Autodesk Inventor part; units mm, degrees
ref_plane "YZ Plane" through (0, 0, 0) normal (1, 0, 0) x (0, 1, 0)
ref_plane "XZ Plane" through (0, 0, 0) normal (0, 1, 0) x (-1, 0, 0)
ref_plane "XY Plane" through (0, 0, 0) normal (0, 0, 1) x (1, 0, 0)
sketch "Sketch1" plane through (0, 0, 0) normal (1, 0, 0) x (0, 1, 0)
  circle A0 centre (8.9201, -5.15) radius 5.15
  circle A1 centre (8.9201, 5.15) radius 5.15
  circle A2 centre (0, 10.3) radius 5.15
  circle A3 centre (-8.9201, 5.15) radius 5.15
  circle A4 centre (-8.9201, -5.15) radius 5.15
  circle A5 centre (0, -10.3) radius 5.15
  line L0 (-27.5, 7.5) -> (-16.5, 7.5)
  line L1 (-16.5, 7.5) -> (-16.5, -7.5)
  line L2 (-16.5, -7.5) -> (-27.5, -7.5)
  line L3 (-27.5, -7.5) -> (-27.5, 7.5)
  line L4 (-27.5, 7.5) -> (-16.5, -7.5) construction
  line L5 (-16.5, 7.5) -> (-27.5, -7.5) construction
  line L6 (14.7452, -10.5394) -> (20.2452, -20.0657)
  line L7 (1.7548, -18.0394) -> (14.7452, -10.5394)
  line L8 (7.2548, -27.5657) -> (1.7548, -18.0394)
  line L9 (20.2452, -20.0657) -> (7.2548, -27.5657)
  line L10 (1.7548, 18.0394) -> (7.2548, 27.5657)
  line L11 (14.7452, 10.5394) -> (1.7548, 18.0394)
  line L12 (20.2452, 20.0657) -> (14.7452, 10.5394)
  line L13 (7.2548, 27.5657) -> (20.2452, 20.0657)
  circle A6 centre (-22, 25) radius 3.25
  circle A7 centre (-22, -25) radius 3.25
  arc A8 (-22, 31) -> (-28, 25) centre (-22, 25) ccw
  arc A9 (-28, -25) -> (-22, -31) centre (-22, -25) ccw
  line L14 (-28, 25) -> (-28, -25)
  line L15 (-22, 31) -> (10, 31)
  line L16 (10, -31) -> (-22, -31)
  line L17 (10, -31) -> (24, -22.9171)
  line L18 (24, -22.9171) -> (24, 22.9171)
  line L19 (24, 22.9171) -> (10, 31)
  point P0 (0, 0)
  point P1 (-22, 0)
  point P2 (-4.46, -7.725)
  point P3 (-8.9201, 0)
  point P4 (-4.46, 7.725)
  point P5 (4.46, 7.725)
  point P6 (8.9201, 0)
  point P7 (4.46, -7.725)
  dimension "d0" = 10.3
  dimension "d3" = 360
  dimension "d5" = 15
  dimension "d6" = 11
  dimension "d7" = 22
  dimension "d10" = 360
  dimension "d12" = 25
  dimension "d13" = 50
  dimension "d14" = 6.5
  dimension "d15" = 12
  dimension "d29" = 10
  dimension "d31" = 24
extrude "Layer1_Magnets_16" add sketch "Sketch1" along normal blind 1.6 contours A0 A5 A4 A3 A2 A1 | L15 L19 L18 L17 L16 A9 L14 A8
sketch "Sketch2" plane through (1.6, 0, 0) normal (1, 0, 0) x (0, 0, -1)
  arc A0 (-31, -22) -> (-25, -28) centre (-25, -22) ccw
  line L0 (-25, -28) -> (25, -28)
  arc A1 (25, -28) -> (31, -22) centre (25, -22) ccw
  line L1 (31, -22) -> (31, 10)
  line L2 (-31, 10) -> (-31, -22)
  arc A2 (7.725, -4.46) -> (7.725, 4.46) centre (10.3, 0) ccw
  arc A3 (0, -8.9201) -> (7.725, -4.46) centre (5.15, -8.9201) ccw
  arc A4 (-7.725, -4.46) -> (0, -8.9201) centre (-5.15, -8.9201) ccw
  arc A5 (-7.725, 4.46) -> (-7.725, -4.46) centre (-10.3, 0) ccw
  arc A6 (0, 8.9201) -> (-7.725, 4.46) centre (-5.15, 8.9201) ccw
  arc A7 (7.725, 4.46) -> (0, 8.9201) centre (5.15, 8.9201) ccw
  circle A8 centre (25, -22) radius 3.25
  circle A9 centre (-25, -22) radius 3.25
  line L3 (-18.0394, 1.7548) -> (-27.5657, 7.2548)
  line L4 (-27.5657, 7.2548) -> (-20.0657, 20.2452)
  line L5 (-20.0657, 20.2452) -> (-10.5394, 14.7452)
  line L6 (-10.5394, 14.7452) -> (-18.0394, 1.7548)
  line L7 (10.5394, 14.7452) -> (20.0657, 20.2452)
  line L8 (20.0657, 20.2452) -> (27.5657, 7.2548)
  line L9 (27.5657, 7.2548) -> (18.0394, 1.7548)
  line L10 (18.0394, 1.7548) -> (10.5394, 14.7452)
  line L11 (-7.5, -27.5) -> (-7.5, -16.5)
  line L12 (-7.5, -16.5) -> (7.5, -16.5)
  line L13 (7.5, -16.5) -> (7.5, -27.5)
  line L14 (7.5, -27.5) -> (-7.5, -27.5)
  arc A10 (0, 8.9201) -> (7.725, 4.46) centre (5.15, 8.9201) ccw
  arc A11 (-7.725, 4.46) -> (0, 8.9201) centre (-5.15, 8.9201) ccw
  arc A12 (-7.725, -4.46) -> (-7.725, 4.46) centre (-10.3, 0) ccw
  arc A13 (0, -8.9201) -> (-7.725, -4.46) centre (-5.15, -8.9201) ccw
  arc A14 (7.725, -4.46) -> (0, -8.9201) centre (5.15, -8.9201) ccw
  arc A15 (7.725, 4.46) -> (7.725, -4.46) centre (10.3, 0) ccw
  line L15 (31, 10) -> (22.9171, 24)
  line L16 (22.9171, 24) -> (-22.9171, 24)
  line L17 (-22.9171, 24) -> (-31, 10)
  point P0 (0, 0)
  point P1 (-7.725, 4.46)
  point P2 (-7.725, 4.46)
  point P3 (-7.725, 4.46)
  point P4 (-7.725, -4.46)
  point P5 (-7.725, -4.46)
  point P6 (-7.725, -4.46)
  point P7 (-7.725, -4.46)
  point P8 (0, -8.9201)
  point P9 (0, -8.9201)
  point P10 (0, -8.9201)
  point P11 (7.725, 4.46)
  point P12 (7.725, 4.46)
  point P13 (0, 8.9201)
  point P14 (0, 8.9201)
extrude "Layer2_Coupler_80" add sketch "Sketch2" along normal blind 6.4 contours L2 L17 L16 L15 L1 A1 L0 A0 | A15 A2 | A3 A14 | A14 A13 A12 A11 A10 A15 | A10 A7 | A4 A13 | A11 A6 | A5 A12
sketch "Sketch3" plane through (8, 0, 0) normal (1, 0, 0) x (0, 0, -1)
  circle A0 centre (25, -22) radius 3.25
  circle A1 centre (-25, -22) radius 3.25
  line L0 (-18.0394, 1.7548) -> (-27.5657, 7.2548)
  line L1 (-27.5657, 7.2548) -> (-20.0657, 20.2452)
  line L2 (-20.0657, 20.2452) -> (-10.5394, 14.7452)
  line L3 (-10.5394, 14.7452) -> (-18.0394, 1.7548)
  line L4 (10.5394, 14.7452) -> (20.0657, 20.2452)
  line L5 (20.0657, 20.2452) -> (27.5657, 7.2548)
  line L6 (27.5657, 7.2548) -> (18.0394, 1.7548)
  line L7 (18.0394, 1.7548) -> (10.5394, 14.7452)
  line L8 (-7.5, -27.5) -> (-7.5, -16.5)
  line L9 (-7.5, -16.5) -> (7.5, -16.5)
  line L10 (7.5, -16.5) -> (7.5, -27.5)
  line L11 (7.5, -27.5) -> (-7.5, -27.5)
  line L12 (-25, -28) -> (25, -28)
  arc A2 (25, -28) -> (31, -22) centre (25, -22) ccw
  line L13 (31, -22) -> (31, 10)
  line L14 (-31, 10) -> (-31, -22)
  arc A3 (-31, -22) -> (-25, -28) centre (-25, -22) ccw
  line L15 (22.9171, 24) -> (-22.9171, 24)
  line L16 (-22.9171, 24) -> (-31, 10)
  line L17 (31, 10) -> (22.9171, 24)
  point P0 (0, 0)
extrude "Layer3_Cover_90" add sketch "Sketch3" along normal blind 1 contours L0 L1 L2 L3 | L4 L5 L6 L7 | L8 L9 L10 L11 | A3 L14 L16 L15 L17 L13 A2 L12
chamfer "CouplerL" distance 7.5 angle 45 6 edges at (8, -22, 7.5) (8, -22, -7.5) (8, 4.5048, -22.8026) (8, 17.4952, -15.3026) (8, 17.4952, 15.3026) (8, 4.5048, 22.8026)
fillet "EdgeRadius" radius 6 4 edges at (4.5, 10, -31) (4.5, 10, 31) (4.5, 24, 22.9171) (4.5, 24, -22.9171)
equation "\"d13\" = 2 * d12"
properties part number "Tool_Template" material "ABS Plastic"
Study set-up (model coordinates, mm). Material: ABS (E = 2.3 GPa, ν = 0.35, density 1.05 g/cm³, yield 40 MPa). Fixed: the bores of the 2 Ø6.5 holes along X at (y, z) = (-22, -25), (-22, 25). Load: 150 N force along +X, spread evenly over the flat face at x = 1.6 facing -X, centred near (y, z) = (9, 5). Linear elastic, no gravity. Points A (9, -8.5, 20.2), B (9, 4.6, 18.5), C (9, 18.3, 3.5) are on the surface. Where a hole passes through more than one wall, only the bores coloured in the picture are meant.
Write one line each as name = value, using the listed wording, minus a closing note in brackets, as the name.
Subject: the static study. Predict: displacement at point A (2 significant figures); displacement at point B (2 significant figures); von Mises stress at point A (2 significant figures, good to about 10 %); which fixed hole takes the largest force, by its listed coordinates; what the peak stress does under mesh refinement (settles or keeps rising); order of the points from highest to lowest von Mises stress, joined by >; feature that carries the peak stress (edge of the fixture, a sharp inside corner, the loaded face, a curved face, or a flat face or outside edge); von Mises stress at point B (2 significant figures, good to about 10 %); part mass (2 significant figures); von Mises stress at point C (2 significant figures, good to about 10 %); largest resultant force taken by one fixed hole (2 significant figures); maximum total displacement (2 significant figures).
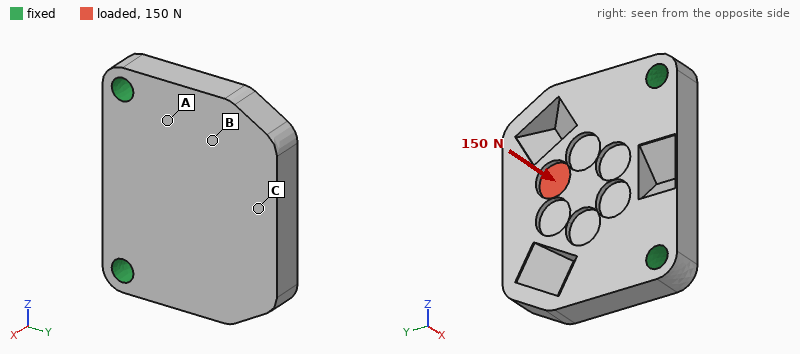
displacement at point A = 0.091 mm
displacement at point B = 0.24 mm
von Mises stress at point A = 4.3 MPa
which fixed hole takes the largest force, by its listed coordinates = (-22, 25)
what the peak stress does under mesh refinement = keeps rising
order of the points from highest to lowest von Mises stress, joined by > = A > C > B
feature that carries the peak stress = edge of the fixture
von Mises stress at point B = 1.2 MPa
part mass = 26 g
von Mises stress at point C = 2.6 MPa
largest resultant force taken by one fixed hole = 91 N
maximum total displacement = 0.51 mm
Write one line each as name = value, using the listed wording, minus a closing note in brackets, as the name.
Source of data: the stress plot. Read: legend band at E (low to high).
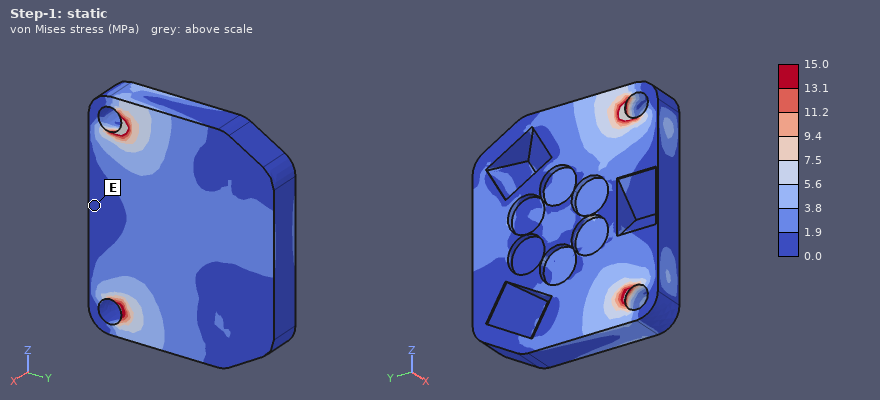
legend band at E = 0.0 to 1.9 MPa
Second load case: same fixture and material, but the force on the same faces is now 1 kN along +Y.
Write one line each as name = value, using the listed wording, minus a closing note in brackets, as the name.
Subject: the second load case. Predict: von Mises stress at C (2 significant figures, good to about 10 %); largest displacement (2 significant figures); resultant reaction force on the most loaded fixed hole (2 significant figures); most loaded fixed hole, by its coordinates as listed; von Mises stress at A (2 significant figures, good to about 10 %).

von Mises stress at C = 5.0 MPa
largest displacement = 0.56 mm
resultant reaction force on the most loaded fixed hole = 640 N
most loaded fixed hole, by its coordinates as listed = (-22, 25)
von Mises stress at A = 3.0 MPa
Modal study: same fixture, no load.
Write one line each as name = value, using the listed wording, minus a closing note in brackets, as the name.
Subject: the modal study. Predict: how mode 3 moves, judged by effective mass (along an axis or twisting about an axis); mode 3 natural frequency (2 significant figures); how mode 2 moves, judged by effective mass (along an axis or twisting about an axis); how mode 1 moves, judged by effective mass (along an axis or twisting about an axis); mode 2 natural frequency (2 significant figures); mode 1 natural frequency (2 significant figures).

how mode 3 moves, judged by effective mass = along Z
mode 3 natural frequency = 4000 Hz
how mode 2 moves, judged by effective mass = twisting about Y
how mode 1 moves, judged by effective mass = along X
mode 2 natural frequency = 2100 Hz
mode 1 natural frequency = 930 Hz
